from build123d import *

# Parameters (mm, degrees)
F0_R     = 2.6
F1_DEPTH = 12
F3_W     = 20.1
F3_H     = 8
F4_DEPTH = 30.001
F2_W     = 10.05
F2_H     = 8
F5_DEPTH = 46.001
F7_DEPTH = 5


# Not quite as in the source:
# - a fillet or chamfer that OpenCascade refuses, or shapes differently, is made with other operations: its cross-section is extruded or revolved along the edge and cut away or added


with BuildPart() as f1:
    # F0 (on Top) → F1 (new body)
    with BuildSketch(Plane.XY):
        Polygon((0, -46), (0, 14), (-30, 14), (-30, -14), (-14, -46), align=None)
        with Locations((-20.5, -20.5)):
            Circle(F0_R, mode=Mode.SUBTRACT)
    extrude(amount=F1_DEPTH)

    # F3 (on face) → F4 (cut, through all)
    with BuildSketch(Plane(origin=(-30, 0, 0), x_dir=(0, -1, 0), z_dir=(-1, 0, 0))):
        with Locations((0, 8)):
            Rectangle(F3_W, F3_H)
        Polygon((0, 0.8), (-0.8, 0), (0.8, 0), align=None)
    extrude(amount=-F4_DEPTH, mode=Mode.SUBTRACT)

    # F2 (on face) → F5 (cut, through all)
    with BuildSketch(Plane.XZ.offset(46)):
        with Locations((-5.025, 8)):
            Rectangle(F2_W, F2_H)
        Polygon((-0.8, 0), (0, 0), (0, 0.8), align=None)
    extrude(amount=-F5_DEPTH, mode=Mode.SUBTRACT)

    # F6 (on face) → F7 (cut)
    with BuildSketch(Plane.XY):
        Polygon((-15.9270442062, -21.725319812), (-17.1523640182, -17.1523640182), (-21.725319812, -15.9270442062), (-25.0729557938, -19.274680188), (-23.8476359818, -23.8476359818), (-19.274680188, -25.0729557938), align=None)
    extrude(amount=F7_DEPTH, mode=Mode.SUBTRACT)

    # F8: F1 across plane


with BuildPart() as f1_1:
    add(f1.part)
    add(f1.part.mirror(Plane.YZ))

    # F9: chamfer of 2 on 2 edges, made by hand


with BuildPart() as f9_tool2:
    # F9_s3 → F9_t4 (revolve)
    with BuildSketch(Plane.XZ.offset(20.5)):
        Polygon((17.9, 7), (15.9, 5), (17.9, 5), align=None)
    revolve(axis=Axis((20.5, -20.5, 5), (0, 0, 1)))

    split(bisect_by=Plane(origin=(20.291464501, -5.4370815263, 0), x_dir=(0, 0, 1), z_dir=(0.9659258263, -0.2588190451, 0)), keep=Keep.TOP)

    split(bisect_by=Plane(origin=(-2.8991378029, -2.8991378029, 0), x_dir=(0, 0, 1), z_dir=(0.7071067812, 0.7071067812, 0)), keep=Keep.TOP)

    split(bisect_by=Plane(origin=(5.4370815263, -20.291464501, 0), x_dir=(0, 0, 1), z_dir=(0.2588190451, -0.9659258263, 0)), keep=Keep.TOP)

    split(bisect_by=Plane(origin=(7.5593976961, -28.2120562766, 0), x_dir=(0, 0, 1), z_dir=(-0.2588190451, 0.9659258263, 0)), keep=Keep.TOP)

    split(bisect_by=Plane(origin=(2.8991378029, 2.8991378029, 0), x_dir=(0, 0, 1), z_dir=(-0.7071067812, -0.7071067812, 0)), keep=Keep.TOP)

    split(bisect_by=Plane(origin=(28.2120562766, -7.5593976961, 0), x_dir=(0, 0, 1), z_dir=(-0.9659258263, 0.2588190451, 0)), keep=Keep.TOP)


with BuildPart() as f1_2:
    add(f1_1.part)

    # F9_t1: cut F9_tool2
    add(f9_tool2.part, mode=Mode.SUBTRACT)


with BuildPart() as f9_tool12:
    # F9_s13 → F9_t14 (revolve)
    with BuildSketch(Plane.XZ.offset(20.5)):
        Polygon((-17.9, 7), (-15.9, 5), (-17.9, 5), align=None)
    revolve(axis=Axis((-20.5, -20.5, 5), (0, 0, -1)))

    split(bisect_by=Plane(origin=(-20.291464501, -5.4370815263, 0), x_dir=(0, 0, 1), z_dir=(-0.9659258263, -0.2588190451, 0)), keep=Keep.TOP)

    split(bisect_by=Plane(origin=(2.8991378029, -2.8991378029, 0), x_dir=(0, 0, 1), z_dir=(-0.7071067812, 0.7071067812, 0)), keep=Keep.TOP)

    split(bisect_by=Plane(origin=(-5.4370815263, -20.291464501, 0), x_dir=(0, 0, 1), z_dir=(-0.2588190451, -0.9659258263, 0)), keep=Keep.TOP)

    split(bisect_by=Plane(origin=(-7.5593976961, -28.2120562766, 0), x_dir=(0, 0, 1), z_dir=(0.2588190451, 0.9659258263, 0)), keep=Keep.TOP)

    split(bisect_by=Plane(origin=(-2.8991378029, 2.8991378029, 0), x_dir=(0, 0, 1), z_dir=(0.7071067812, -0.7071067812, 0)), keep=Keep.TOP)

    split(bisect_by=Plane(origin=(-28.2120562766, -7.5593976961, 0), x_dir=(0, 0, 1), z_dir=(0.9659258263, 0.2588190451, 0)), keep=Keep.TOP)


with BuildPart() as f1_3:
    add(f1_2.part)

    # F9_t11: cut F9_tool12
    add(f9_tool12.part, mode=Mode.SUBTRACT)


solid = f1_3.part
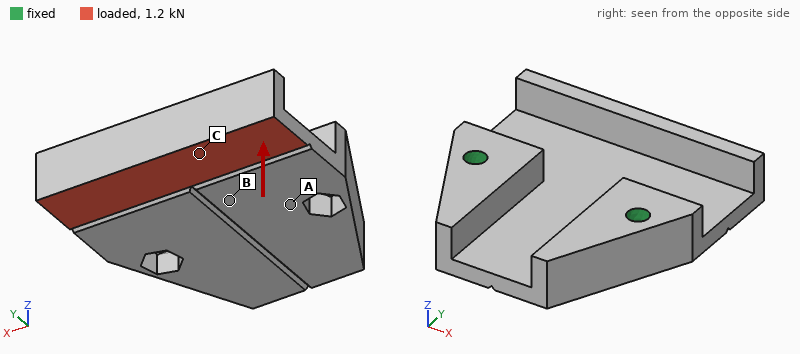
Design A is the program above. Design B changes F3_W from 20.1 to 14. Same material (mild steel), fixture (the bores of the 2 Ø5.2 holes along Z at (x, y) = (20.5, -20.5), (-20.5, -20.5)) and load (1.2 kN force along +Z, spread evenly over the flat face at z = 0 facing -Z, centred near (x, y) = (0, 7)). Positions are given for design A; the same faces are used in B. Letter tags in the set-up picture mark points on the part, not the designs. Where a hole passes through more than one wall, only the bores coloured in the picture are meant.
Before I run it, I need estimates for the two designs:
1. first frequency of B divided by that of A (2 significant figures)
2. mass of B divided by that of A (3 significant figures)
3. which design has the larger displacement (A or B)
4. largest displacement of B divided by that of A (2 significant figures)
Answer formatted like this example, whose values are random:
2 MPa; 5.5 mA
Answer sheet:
1.0; 1.12; A; 0.76
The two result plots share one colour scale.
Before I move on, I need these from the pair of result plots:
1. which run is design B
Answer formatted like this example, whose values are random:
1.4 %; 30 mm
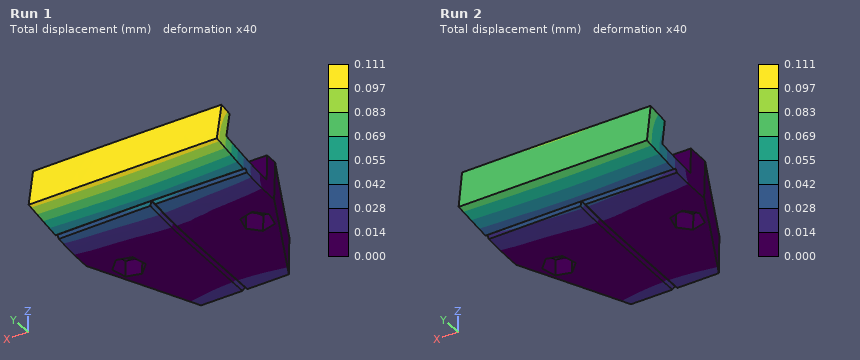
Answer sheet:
Run 2
